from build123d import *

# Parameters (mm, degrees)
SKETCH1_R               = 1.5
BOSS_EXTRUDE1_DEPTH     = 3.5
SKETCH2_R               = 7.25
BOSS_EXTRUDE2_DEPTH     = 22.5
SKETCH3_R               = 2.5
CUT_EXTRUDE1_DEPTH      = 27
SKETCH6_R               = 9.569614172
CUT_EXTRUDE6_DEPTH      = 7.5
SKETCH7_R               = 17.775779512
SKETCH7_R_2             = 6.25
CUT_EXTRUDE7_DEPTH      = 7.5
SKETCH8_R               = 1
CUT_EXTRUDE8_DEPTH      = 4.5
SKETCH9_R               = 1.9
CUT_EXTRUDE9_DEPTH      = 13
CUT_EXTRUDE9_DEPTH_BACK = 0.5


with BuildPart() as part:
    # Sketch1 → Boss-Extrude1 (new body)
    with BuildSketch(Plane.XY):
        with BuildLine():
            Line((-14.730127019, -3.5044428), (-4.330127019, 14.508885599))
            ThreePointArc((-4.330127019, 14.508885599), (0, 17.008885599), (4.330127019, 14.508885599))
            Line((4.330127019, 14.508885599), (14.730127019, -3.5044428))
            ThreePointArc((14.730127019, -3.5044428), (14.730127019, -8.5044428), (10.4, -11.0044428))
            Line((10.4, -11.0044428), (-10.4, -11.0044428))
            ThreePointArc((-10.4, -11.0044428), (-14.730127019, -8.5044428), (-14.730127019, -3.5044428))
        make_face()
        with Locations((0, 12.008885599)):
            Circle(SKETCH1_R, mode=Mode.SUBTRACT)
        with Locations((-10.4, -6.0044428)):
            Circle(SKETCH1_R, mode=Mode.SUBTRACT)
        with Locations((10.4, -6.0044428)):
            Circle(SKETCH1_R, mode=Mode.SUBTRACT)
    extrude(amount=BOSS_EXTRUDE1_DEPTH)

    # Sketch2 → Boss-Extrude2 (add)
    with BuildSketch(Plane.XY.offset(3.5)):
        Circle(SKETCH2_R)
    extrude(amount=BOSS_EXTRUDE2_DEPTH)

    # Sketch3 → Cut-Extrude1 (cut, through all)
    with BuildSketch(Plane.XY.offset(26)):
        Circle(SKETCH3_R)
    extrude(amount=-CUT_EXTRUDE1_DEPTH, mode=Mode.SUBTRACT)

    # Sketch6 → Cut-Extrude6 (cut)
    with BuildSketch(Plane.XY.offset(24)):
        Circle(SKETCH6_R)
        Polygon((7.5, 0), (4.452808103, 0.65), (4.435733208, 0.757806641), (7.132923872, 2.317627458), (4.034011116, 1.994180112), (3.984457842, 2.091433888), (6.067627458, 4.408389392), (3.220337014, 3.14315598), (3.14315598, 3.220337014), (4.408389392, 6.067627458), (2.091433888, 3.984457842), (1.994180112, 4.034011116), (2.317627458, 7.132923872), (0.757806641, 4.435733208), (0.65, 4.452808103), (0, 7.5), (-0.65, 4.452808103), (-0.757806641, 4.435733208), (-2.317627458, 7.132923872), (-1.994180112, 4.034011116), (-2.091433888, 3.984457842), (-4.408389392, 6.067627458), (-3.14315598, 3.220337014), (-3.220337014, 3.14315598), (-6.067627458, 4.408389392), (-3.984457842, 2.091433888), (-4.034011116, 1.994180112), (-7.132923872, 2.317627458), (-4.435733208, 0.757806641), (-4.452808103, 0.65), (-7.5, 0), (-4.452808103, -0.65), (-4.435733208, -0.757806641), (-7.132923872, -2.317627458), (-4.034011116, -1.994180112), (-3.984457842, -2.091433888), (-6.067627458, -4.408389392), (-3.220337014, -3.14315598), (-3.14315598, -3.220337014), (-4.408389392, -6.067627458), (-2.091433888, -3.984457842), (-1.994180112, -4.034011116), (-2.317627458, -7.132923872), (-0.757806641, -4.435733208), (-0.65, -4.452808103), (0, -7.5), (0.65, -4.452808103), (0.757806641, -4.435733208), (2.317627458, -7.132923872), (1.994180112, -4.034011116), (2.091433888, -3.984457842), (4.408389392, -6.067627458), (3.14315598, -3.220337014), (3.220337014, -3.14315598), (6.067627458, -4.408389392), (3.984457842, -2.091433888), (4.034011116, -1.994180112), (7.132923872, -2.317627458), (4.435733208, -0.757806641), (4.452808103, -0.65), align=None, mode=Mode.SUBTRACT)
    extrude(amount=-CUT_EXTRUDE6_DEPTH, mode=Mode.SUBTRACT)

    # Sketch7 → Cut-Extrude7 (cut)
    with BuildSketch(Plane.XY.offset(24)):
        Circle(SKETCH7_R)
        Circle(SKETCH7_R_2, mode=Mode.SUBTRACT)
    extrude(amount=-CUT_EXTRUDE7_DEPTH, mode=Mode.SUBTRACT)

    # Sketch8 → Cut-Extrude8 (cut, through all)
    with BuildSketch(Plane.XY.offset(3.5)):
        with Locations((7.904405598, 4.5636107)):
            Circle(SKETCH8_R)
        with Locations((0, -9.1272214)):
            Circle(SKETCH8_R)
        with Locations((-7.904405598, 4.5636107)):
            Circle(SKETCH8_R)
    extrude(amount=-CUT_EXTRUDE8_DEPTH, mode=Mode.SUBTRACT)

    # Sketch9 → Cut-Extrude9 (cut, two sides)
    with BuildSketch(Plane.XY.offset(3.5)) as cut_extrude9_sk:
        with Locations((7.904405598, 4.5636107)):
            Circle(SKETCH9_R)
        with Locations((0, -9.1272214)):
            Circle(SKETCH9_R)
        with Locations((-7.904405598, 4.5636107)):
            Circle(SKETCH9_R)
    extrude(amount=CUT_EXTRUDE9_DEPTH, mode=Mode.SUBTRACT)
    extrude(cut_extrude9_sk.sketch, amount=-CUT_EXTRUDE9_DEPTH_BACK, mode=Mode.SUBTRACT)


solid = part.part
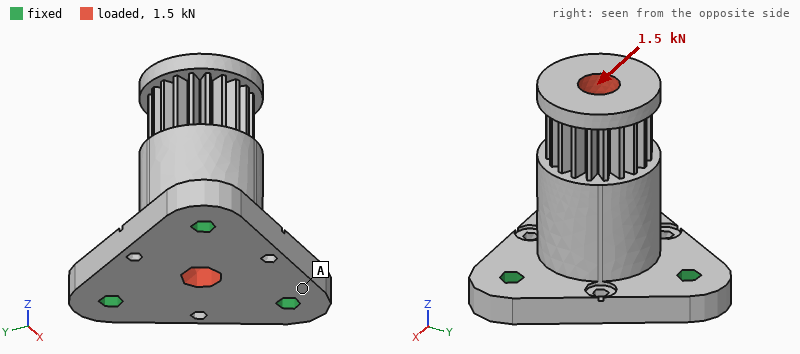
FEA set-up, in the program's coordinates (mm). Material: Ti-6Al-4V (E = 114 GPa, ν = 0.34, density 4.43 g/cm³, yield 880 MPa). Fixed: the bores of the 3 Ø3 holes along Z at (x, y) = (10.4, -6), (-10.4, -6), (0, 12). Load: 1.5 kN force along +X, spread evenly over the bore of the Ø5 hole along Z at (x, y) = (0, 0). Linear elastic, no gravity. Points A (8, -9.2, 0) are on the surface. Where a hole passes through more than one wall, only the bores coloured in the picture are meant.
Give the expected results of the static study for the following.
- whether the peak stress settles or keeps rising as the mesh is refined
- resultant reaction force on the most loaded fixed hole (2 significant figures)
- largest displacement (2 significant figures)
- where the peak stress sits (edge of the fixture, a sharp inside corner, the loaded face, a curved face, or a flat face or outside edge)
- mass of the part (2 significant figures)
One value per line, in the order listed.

keeps rising
1.1 kN
38 µm
edge of the fixture
20 g
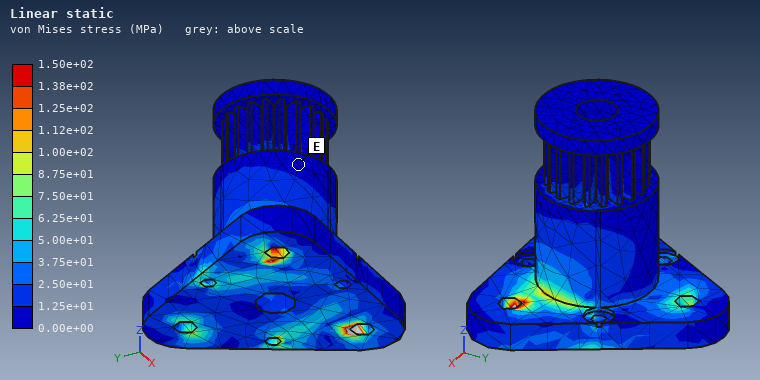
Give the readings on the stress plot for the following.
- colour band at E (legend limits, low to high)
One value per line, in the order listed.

0.00e+00 to 1.25e+01 MPa
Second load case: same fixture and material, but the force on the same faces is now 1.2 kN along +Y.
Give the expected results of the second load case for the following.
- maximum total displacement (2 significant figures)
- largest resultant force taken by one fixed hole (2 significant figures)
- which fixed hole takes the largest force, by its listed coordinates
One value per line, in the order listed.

31 µm
1.0 kN
(0, 12)
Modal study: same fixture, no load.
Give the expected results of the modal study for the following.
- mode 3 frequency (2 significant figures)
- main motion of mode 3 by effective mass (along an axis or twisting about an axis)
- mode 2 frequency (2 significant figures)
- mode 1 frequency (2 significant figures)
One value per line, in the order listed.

22 kHz
along Z
11 kHz
11 kHz
